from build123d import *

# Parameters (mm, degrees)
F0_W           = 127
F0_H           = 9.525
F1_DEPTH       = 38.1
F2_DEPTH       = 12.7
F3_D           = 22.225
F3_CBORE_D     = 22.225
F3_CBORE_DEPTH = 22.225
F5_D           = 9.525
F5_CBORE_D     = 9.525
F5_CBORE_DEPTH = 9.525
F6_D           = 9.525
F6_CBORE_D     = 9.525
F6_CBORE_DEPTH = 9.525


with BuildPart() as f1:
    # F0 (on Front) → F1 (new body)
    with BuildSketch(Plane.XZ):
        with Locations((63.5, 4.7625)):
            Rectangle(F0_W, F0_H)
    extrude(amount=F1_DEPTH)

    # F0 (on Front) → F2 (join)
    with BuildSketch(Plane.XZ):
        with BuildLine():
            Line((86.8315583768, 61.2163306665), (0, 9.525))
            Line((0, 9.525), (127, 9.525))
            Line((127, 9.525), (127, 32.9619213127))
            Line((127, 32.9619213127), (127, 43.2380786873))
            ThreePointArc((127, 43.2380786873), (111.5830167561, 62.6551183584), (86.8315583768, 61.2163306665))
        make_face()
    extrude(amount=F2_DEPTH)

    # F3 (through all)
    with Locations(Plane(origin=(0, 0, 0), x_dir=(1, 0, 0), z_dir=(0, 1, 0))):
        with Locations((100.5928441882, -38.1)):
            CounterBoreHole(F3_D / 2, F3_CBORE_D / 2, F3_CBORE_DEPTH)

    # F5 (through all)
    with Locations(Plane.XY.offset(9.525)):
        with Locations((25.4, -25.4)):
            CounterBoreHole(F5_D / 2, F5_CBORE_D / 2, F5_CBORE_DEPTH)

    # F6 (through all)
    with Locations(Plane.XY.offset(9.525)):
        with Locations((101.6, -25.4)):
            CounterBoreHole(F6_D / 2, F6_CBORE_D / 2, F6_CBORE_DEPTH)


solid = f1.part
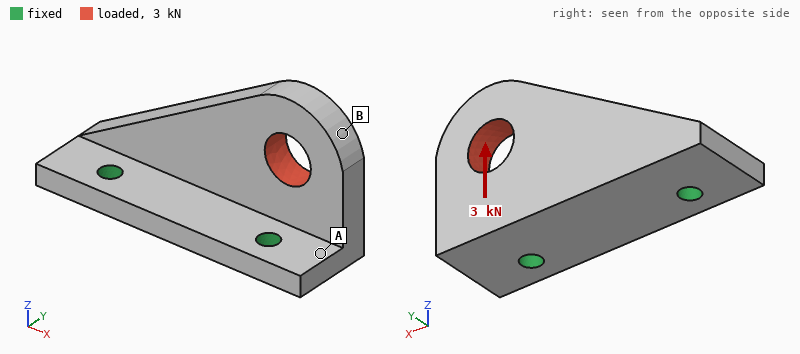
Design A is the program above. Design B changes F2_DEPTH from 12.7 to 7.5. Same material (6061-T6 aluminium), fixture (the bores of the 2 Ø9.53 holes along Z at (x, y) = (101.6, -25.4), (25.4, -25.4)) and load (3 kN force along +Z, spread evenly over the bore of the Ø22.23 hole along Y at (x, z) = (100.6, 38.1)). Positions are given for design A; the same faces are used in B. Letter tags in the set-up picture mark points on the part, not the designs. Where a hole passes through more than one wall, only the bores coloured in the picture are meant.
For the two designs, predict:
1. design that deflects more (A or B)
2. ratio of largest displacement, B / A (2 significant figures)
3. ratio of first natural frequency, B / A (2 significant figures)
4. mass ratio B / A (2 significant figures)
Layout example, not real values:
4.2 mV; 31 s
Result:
B; 1.4; 0.93; 0.78
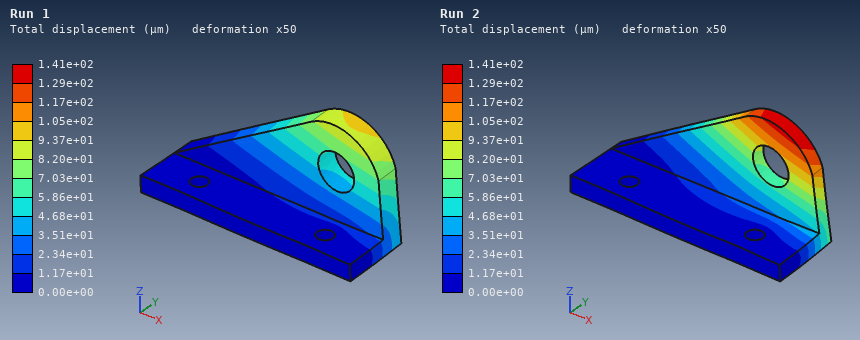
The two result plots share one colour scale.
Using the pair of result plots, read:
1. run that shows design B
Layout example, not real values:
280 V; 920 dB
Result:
Run 2
